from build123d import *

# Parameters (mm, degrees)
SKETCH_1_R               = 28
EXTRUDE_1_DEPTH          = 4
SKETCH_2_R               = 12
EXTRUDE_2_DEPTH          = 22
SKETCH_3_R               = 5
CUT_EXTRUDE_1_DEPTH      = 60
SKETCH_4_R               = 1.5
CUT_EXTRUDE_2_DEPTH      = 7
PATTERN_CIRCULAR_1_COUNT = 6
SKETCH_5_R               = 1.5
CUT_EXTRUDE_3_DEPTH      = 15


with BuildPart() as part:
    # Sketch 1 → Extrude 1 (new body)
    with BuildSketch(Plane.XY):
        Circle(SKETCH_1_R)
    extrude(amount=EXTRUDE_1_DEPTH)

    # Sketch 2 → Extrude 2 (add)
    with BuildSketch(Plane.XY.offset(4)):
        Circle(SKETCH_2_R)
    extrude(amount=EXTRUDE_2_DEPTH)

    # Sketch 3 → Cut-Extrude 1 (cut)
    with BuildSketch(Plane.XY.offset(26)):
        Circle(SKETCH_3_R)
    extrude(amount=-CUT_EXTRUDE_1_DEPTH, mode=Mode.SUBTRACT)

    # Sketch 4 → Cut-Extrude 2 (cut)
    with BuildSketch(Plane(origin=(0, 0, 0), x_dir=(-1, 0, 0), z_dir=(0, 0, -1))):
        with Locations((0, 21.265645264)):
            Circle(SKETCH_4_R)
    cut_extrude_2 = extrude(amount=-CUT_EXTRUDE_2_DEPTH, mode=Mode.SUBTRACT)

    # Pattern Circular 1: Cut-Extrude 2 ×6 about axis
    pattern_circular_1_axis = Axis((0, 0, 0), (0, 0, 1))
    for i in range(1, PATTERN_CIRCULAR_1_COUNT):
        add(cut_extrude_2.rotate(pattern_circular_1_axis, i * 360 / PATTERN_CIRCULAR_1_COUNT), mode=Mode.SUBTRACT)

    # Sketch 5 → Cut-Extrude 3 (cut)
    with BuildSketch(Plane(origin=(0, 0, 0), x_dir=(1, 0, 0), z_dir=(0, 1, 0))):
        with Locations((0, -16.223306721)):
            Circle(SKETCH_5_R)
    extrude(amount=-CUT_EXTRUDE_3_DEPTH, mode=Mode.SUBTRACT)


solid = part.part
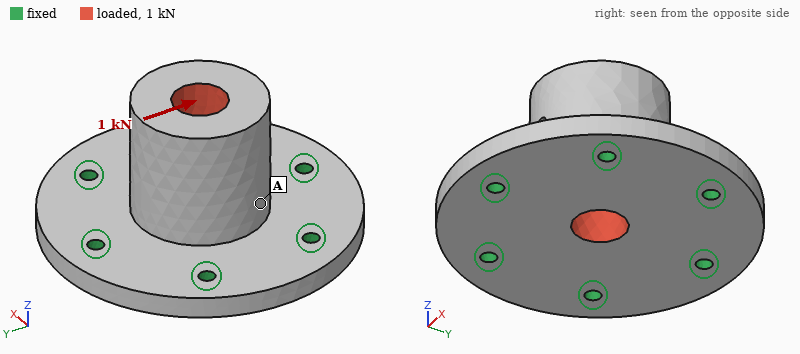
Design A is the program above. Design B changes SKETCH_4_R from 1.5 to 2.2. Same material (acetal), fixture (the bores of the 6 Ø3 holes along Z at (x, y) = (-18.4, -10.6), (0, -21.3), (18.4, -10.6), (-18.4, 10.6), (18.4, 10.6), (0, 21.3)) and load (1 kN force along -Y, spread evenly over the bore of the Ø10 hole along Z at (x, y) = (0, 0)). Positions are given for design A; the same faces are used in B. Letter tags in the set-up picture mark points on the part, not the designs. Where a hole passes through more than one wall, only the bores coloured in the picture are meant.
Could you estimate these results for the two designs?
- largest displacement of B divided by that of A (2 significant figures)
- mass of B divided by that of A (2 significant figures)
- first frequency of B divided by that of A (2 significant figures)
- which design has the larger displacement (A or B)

0.90
0.99
1.1
A
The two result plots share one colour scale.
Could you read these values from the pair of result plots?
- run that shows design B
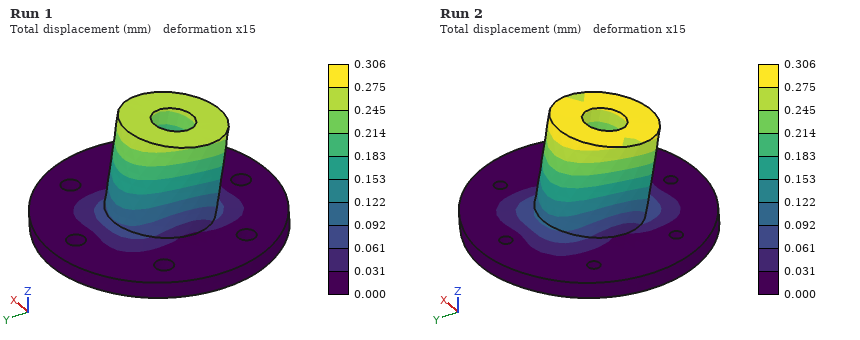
Run 1
